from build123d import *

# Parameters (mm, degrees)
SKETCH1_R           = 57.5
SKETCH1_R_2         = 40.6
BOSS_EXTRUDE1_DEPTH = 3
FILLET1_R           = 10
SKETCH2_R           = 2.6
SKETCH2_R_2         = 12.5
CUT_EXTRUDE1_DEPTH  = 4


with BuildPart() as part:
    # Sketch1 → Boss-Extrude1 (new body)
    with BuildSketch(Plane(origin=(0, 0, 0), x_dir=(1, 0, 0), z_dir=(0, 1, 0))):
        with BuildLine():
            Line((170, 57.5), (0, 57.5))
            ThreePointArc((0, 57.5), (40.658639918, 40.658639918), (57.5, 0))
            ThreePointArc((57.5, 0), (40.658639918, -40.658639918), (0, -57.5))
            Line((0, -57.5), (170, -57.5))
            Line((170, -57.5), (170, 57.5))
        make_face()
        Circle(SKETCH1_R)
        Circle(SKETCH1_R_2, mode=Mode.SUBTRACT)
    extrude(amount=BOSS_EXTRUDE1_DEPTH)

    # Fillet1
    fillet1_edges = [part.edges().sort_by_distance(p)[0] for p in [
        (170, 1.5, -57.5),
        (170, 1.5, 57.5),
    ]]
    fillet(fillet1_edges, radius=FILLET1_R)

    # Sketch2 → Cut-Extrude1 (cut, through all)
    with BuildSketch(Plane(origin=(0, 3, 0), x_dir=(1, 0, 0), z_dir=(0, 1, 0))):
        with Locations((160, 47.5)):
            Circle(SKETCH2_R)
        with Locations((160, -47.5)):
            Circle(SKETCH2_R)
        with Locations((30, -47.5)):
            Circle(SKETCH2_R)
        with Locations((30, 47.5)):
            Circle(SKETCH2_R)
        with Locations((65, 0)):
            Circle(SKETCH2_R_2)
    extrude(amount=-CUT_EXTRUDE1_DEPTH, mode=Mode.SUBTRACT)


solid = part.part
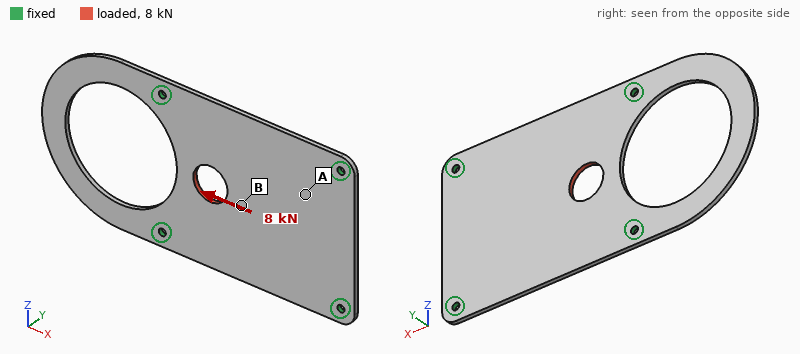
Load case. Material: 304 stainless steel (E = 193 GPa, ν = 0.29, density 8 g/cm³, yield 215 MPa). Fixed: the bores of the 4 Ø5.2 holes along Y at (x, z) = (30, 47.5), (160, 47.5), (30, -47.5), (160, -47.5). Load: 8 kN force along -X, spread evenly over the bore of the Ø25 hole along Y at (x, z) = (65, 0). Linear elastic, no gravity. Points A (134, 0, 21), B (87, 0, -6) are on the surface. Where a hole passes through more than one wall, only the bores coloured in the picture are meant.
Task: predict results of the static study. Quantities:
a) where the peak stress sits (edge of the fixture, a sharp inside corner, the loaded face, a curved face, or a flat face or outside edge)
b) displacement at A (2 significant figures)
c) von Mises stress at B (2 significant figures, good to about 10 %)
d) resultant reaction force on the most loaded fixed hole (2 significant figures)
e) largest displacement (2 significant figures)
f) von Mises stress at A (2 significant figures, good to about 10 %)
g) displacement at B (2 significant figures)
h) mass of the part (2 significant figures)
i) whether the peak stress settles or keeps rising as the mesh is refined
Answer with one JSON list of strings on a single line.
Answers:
["edge of the fixture", "4.6 µm", "31 MPa", "2.7 kN", "18 µm", "12 MPa", "8.7 µm", "450 g", "keeps rising"]
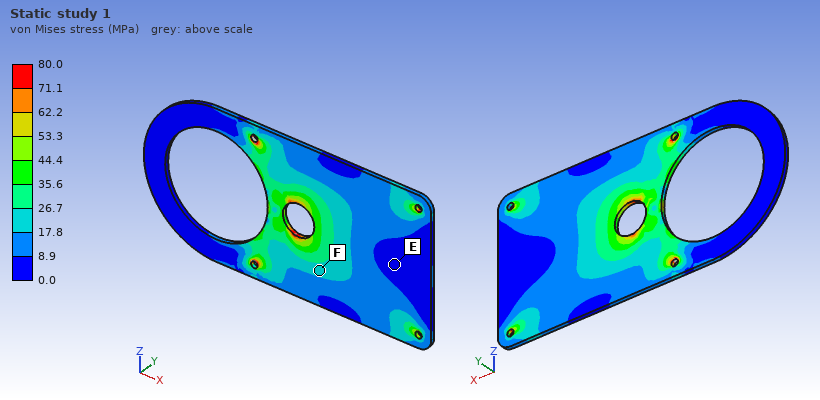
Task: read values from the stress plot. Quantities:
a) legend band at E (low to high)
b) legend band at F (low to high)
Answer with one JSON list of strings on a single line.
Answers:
["0.0 to 8.9 MPa", "17.8 to 26.7 MPa"]
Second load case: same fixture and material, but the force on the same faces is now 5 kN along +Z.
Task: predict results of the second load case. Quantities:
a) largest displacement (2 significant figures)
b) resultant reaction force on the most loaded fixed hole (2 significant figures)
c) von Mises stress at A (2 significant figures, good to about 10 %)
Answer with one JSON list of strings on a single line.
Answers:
["11 µm", "1.7 kN", "11 MPa"]
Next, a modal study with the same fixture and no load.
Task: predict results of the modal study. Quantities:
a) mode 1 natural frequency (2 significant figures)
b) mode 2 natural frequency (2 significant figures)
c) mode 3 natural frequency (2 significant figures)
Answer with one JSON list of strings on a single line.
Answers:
["270 Hz", "710 Hz", "740 Hz"]
